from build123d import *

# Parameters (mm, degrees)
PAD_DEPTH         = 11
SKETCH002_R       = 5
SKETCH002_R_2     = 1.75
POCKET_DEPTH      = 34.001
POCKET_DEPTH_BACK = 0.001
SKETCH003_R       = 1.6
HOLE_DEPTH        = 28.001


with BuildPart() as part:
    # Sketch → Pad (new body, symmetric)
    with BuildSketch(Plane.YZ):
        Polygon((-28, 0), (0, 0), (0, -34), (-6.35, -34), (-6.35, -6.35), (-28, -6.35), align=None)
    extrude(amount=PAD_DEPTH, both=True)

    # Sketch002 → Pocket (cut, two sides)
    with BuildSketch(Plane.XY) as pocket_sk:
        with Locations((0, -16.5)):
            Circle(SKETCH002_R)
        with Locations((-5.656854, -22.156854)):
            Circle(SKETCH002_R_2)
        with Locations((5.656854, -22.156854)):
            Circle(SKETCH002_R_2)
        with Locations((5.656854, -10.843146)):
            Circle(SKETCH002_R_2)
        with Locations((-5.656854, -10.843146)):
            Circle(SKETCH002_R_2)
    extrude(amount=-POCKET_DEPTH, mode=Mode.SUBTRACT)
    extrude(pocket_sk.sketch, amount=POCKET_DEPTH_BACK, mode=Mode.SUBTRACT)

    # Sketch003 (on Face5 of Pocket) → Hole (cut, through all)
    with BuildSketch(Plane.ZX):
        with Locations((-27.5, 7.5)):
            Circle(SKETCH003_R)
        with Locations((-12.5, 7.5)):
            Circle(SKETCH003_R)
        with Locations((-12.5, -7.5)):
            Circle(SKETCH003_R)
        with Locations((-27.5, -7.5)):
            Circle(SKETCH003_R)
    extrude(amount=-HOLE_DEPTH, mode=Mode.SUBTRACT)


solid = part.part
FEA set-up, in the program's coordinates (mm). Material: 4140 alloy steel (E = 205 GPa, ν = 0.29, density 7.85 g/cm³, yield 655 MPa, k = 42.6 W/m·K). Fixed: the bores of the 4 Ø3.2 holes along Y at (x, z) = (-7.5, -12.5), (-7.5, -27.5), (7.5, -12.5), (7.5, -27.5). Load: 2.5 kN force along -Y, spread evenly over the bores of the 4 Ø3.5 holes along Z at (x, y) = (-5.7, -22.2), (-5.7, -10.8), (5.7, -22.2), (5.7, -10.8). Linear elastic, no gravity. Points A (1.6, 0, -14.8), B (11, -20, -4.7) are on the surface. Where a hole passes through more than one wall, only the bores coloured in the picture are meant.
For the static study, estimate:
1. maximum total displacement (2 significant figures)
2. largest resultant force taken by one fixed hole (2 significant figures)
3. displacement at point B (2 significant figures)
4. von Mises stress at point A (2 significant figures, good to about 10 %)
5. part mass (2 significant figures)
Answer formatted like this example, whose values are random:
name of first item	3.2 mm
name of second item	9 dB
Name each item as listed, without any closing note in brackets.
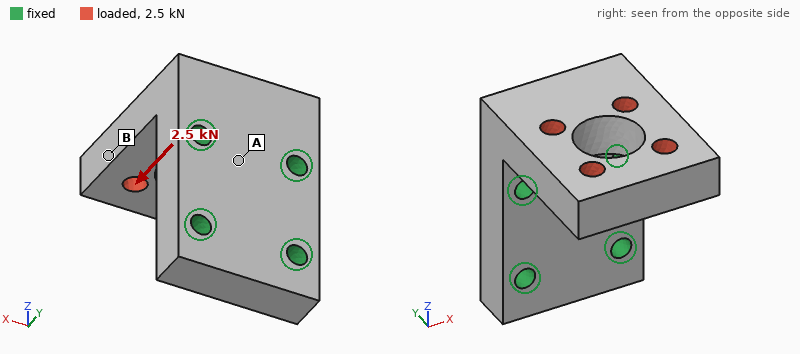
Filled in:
maximum total displacement	34 µm
largest resultant force taken by one fixed hole	1.4 kN
displacement at point B	22 µm
von Mises stress at point A	41 MPa
part mass	54 g
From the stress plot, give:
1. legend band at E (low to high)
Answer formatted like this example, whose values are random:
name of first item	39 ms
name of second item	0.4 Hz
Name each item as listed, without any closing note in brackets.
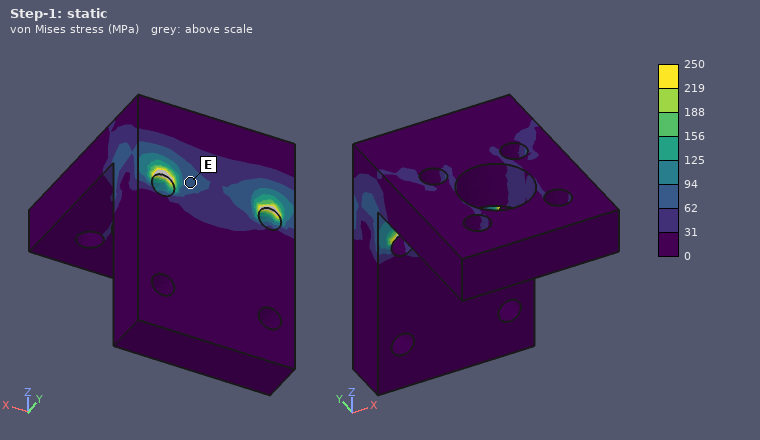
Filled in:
legend band at E	62 to 94 MPa
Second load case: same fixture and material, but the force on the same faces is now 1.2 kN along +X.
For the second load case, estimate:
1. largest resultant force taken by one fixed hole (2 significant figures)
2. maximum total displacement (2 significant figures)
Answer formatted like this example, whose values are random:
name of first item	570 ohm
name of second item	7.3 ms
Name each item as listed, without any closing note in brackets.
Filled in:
largest resultant force taken by one fixed hole	1.2 kN
maximum total displacement	19 µm
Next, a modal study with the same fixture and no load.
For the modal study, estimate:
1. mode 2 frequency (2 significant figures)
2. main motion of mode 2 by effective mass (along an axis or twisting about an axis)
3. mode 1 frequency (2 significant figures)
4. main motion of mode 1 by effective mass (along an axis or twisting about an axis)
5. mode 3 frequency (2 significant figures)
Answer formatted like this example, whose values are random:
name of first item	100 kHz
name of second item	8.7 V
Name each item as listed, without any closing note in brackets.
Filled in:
mode 2 frequency	10 kHz
main motion of mode 2 by effective mass	along X
mode 1 frequency	5500 Hz
main motion of mode 1 by effective mass	along Z
mode 3 frequency	15 kHz
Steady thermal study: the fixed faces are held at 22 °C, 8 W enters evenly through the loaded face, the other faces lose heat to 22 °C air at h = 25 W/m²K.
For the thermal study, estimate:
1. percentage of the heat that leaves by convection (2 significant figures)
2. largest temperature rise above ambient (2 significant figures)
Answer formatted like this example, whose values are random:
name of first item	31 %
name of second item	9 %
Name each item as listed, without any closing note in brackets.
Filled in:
percentage of the heat that leaves by convection	12 %
largest temperature rise above ambient	33 K
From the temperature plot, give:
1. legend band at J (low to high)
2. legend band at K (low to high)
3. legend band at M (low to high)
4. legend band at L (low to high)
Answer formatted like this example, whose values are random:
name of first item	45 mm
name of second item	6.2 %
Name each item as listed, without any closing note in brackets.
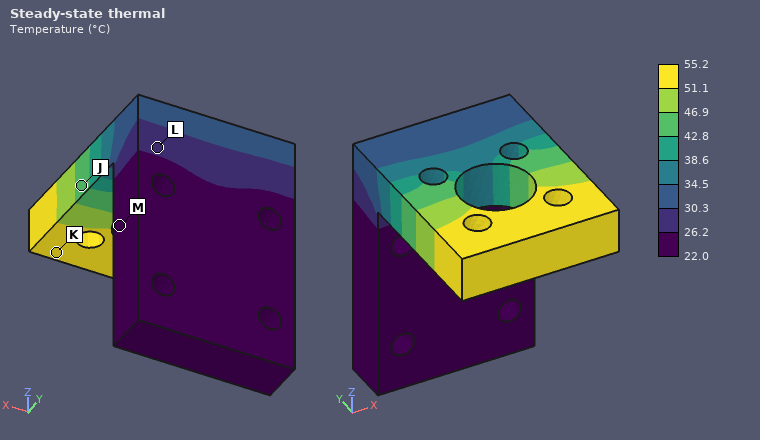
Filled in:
legend band at J	42.8 to 46.9 °C
legend band at K	51.1 to 55.2 °C
legend band at M	22.0 to 26.2 °C
legend band at L	26.2 to 30.3 °C
